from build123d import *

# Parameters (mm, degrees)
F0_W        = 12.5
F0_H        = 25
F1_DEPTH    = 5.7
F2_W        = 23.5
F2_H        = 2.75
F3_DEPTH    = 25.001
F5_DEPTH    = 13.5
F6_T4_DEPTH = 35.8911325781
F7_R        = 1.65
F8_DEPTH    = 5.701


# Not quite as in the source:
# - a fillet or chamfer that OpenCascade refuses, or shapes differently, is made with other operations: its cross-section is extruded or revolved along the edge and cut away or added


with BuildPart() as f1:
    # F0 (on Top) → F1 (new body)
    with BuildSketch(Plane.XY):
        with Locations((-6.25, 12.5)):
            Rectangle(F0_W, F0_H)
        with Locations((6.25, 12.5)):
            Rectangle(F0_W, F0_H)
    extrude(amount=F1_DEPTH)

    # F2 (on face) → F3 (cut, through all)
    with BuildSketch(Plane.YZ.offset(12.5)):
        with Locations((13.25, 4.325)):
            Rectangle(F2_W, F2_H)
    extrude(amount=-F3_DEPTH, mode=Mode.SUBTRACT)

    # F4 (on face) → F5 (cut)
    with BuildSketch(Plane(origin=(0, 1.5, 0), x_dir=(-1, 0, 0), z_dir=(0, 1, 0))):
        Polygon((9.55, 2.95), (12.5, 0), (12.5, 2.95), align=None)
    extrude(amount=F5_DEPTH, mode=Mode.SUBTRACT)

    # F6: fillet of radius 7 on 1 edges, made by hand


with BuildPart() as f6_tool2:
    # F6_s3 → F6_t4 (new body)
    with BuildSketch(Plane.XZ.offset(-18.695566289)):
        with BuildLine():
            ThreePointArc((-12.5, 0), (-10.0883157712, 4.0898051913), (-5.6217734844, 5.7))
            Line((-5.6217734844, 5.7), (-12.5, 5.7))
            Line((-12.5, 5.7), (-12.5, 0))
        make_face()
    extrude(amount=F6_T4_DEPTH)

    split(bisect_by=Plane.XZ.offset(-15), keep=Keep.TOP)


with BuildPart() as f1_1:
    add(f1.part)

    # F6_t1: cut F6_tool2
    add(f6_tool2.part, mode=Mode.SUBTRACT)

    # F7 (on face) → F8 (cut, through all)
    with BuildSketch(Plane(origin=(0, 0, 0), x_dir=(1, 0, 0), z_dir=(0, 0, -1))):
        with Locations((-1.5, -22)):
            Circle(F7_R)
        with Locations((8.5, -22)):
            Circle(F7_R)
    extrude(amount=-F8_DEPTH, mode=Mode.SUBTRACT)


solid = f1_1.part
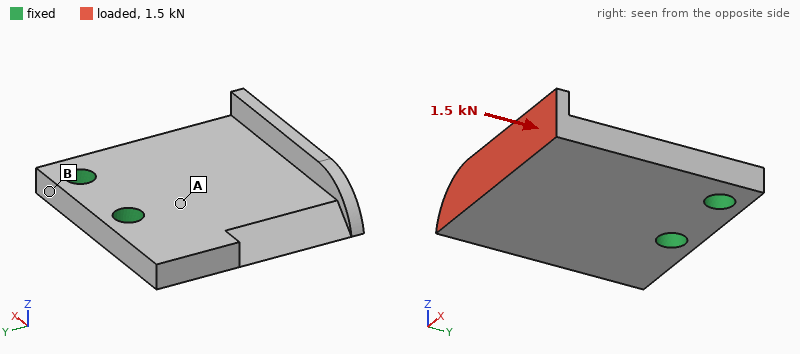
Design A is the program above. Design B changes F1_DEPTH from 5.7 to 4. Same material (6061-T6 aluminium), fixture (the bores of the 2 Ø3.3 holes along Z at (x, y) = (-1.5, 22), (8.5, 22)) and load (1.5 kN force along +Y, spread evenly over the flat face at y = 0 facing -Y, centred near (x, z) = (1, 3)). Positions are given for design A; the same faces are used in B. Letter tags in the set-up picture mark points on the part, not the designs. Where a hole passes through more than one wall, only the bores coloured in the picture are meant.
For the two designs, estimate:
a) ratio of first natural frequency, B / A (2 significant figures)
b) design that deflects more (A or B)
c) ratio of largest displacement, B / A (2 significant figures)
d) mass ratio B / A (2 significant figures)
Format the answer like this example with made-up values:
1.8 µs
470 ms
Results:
1.1
A
0.40
0.97
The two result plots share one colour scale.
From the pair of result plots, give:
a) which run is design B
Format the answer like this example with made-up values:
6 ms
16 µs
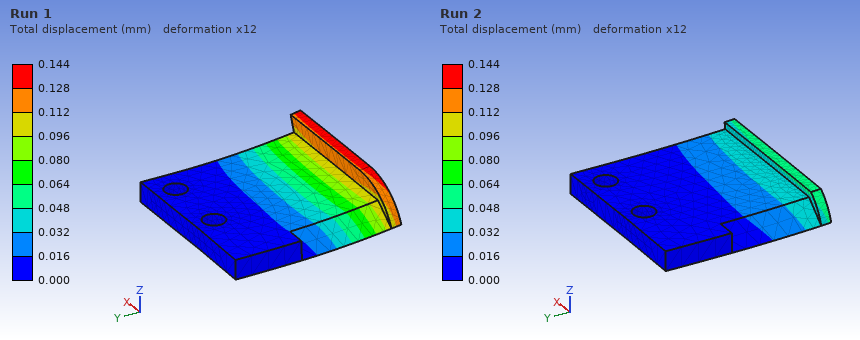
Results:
Run 2
